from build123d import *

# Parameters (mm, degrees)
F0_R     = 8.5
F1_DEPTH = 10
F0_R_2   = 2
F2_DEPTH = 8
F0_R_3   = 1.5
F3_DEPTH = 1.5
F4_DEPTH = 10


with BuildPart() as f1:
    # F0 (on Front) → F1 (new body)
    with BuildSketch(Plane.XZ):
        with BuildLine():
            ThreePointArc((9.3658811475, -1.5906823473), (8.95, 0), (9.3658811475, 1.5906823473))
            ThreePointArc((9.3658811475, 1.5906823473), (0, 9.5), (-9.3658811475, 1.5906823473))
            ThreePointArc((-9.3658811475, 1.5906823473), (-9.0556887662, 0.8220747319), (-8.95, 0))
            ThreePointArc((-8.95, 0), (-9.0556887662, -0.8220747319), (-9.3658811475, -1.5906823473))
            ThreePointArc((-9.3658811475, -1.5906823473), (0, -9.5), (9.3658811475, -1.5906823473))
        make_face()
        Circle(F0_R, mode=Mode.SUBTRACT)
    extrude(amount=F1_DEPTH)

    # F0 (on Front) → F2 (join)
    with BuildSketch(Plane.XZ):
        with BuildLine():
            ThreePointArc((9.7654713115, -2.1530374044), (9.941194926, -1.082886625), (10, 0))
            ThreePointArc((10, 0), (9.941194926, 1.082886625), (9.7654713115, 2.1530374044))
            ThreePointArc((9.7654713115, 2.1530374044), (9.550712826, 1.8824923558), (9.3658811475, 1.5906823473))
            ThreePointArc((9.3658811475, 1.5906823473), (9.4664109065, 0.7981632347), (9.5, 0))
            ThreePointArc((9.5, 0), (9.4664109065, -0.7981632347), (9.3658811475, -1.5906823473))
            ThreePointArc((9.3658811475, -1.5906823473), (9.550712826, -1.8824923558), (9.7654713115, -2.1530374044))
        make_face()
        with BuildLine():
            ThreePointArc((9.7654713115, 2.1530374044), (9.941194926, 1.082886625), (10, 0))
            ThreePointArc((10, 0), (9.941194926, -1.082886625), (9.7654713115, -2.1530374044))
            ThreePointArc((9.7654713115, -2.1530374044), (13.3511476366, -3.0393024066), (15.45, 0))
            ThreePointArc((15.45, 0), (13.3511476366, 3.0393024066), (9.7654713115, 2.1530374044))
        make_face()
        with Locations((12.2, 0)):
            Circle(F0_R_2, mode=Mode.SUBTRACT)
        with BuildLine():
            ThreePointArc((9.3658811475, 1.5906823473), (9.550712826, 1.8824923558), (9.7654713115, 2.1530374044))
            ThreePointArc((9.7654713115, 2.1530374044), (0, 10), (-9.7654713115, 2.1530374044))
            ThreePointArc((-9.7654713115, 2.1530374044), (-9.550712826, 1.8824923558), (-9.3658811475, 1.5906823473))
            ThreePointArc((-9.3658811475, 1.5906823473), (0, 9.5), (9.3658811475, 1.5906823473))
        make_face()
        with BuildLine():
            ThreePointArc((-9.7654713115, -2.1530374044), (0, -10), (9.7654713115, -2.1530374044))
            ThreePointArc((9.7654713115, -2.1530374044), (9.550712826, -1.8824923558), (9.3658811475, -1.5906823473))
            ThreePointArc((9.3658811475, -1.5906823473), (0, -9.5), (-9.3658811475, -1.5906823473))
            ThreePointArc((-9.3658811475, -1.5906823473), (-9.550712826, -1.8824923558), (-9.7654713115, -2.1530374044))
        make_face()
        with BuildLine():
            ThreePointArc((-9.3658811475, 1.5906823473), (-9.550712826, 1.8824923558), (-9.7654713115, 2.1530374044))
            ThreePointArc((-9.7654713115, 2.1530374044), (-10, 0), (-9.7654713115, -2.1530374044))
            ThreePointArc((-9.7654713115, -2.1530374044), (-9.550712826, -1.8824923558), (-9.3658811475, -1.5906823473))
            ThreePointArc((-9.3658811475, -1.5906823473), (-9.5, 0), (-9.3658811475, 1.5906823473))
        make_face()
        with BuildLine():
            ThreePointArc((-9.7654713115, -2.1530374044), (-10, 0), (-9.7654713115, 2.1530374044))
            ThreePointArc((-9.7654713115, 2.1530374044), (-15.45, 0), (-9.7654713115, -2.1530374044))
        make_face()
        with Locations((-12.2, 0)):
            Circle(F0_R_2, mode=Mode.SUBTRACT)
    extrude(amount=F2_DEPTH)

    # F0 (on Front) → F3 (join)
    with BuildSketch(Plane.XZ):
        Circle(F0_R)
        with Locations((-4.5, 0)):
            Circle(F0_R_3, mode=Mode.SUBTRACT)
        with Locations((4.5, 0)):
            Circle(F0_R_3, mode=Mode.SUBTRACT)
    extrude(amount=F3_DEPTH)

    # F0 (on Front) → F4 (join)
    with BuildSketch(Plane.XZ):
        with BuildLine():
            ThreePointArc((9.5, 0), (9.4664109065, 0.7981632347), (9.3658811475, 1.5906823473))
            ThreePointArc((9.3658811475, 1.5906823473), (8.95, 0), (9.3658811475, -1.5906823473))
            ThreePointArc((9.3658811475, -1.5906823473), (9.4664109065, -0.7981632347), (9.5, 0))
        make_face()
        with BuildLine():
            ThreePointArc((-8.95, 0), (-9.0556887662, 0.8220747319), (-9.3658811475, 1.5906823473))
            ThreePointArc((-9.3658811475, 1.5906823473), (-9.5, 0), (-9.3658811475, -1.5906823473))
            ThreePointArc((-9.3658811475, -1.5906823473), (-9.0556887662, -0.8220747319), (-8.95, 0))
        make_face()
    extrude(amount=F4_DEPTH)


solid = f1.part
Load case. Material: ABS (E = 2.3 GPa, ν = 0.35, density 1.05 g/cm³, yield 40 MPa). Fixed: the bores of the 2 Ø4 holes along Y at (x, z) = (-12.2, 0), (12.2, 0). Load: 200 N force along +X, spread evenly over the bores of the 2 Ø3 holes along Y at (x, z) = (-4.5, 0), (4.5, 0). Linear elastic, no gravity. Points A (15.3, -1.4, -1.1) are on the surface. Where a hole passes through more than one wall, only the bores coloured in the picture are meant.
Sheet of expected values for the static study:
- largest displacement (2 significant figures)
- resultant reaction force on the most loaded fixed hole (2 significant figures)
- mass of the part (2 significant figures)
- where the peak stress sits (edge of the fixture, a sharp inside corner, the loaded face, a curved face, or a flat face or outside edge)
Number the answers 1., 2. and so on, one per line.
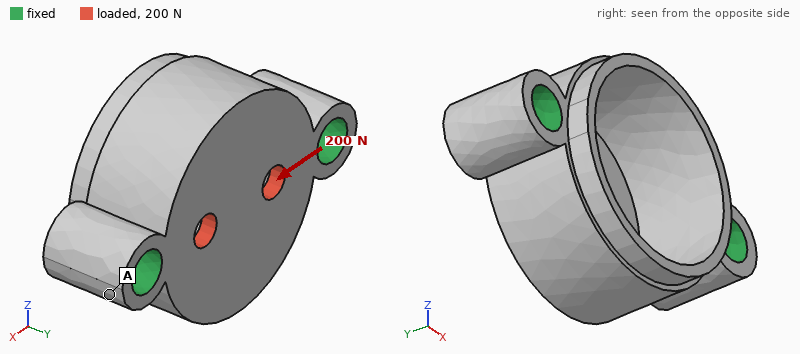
1. 42 µm
2. 100 N
3. 1.5 g
4. the loaded face
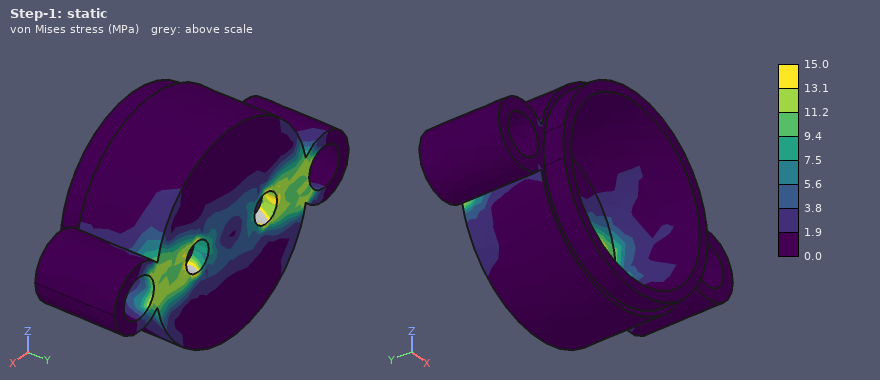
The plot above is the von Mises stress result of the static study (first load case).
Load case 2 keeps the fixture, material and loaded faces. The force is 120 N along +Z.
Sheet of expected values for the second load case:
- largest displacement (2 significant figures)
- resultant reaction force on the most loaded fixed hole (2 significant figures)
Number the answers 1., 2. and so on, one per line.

1. 37 µm
2. 60 N
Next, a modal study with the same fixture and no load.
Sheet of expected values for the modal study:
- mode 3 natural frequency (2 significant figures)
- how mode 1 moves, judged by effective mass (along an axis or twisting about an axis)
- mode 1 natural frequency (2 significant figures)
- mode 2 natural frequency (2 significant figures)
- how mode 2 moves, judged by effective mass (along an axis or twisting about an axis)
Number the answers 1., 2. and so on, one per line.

1. 9100 Hz
2. twisting about X
3. 7900 Hz
4. 8400 Hz
5. along Y
